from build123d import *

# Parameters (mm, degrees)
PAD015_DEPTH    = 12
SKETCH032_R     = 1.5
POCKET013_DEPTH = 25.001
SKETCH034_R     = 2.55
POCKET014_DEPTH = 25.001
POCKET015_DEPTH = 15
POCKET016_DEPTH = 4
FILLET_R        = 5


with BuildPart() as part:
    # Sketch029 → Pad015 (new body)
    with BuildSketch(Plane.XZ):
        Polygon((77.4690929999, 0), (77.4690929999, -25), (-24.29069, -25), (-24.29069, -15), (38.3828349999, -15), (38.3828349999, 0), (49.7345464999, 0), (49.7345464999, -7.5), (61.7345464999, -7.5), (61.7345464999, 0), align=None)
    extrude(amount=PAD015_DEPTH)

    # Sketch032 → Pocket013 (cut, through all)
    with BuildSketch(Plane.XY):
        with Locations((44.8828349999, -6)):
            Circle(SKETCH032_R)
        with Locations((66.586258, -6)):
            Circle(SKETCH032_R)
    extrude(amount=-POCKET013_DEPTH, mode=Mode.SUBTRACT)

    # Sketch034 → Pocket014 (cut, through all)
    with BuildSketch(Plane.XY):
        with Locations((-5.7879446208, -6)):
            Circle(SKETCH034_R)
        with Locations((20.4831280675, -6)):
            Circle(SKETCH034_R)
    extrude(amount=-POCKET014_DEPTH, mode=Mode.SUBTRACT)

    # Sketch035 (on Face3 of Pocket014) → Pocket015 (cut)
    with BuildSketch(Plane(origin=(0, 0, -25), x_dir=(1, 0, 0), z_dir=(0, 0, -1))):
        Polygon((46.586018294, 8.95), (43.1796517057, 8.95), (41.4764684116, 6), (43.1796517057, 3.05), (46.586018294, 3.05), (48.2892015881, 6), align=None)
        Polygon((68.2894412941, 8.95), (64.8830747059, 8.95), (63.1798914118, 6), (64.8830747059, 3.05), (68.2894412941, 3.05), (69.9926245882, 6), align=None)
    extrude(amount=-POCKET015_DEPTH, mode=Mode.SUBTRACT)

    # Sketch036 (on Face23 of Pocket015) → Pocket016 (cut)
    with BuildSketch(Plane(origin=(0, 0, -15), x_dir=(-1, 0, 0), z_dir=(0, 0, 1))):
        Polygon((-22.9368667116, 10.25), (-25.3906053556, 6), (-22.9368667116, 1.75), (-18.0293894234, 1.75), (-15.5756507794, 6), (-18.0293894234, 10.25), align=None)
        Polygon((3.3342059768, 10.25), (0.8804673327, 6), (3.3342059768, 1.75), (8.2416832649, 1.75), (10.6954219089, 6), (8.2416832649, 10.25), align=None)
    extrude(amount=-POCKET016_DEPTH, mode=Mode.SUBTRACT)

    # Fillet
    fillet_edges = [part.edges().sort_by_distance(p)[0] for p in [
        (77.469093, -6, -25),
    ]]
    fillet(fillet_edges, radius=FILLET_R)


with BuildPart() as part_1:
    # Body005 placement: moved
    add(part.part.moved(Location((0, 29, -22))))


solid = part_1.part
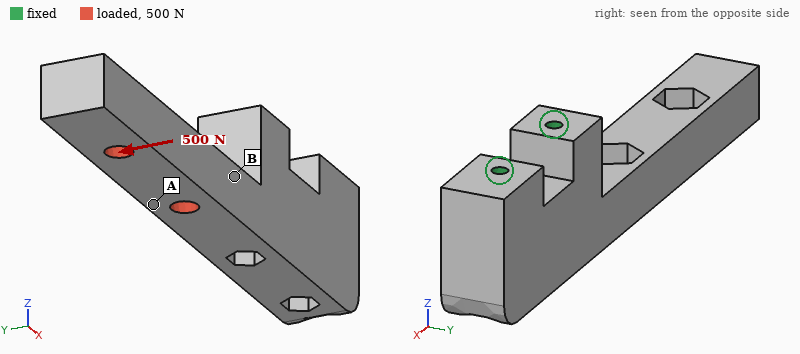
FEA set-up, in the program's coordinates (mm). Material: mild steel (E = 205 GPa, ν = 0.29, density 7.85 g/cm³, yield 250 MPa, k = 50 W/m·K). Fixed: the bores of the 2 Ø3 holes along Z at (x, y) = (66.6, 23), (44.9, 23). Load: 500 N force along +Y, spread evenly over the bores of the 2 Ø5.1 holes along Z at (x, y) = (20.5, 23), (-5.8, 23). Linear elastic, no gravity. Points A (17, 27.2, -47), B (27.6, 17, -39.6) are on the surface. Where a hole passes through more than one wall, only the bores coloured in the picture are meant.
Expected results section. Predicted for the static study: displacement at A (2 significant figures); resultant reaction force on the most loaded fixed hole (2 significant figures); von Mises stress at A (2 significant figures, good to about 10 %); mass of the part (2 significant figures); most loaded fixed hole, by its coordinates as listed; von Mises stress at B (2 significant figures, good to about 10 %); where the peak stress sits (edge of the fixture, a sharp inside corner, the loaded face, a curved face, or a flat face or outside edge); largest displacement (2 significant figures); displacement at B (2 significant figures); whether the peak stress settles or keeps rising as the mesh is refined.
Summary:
0.038 mm
1.1 kN
18 MPa
130 g
(44.9, 23)
47 MPa
edge of the fixture
0.11 mm
0.020 mm
keeps rising
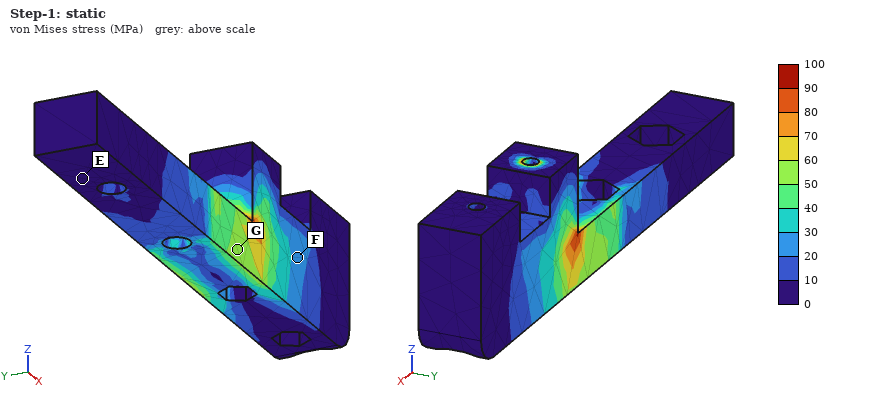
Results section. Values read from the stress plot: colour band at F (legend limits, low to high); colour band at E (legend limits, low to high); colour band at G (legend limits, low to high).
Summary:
20 to 30 MPa
0 to 10 MPa
50 to 60 MPa
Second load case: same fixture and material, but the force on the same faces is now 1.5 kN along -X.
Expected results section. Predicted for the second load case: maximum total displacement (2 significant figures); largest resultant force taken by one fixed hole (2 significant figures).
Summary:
42 µm
1.2 kN
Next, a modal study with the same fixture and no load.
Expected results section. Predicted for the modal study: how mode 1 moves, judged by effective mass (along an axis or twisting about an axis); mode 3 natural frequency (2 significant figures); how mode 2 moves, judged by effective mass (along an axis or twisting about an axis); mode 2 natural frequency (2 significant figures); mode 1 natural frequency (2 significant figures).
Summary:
along Z
8000 Hz
along Y
1700 Hz
1500 Hz
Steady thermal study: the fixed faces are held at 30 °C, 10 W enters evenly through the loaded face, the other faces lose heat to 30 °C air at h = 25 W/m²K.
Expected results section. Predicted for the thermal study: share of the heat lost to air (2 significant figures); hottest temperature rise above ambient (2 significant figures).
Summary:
36 %
57 K
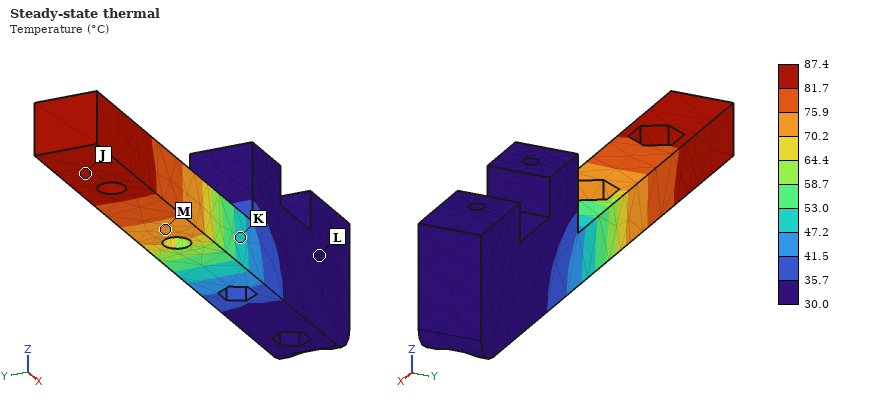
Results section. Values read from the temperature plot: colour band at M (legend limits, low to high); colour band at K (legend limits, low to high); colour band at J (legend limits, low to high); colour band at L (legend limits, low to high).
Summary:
70.2 to 75.9 °C
47.2 to 53.0 °C
81.7 to 87.4 °C
30.0 to 35.7 °C
